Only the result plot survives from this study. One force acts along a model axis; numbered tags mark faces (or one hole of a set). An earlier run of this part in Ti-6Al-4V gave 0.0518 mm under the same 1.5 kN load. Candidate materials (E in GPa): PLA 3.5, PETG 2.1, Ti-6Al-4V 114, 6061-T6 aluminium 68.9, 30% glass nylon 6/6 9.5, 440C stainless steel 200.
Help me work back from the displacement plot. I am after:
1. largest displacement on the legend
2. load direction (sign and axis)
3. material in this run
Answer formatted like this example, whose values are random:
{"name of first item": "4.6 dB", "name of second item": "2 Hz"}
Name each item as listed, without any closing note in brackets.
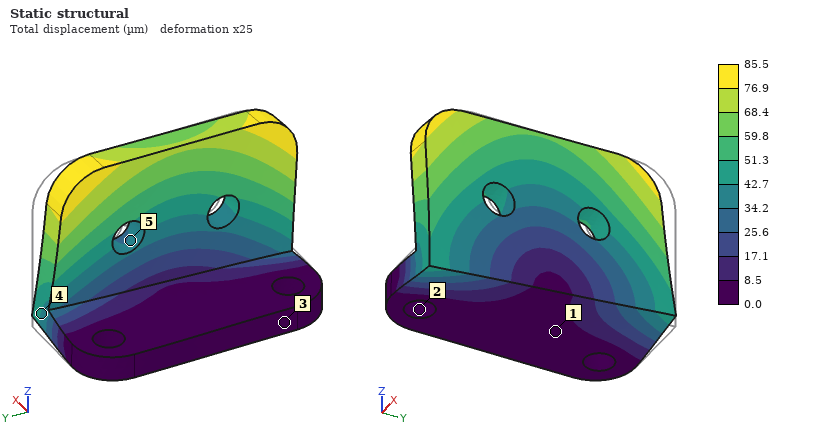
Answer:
{"largest displacement on the legend": "85.5 µm", "load direction": "-Y", "material in this run": "6061-T6 aluminium"}
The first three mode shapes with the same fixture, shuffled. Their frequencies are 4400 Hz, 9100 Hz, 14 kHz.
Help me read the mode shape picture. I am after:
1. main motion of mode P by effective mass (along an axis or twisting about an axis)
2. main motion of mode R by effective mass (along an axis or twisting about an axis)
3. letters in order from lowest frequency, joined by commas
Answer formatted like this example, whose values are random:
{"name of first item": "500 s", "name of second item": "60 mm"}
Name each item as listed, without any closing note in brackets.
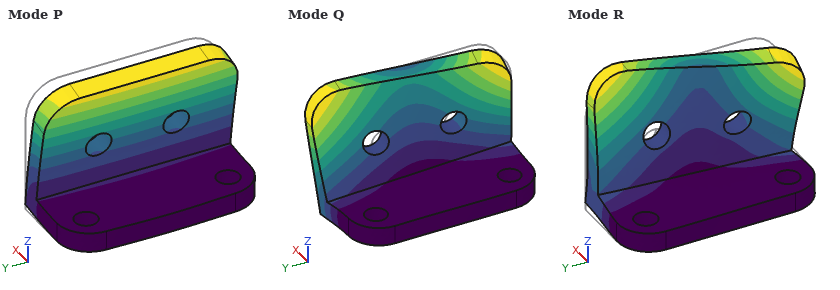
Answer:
{"main motion of mode P by effective mass": "along X", "main motion of mode R by effective mass": "along Y", "letters in order from lowest frequency, joined by commas": "P, Q, R"}
